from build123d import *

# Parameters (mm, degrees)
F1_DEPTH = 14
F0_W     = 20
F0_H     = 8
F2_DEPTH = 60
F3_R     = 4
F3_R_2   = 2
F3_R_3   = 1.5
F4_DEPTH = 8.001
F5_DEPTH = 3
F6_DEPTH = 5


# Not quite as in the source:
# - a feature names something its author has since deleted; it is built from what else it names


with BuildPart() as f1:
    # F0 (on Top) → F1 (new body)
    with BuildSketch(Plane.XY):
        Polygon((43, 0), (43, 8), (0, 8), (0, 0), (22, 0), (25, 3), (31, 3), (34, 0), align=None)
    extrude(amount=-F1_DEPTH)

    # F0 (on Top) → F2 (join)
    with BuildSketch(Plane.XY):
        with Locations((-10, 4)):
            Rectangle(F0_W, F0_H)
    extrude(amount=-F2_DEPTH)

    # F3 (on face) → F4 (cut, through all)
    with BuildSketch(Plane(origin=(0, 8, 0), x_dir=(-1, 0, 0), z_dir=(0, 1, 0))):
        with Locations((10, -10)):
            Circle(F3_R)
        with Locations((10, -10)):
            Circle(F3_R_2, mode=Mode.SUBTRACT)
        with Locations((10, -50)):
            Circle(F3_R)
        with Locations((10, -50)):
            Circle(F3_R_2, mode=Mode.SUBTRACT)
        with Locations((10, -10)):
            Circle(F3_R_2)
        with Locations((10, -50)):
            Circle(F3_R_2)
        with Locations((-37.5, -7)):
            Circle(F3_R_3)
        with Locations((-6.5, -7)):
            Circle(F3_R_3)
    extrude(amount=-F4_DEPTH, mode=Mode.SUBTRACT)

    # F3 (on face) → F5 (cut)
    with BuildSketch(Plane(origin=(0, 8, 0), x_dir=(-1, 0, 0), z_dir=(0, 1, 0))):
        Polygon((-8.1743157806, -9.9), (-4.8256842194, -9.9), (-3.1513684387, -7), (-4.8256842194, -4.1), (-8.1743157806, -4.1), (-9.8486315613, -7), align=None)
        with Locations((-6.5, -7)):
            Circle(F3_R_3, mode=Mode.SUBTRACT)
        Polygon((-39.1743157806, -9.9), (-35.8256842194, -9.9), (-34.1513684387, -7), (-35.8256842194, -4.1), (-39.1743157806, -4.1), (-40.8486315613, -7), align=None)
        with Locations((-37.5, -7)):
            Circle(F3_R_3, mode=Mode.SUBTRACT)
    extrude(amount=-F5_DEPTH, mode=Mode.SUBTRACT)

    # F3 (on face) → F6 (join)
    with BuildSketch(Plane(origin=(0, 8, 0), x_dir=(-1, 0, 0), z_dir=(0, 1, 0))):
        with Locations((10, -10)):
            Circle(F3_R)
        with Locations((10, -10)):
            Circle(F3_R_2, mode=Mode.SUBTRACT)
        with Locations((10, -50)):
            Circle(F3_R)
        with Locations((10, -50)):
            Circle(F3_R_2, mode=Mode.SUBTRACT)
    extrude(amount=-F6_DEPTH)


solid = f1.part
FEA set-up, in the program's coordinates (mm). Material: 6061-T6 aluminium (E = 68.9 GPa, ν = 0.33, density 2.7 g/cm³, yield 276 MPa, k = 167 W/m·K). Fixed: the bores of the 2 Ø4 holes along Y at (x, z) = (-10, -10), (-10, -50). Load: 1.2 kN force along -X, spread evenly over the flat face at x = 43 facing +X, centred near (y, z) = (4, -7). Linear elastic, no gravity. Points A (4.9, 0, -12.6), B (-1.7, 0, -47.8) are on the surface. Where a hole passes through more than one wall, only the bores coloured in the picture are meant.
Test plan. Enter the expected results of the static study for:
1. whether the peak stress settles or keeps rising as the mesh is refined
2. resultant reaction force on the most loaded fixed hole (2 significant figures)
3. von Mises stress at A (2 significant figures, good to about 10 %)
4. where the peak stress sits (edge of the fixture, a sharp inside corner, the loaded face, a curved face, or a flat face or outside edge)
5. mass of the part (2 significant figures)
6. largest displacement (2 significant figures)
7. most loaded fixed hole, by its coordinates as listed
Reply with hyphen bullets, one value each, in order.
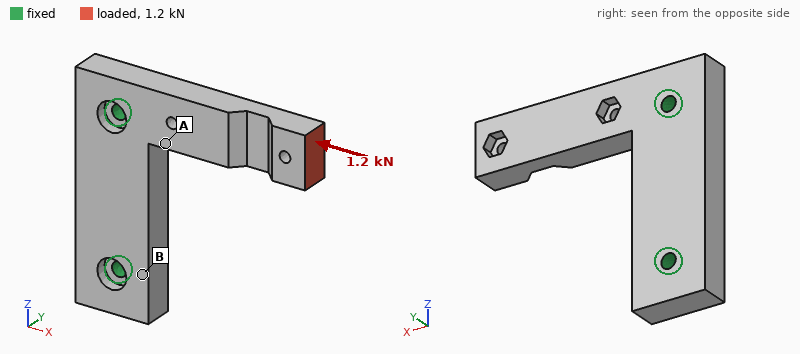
- keeps rising
- 1.3 kN
- 9.7 MPa
- edge of the fixture
- 36 g
- 47 µm
- (-10, -10)
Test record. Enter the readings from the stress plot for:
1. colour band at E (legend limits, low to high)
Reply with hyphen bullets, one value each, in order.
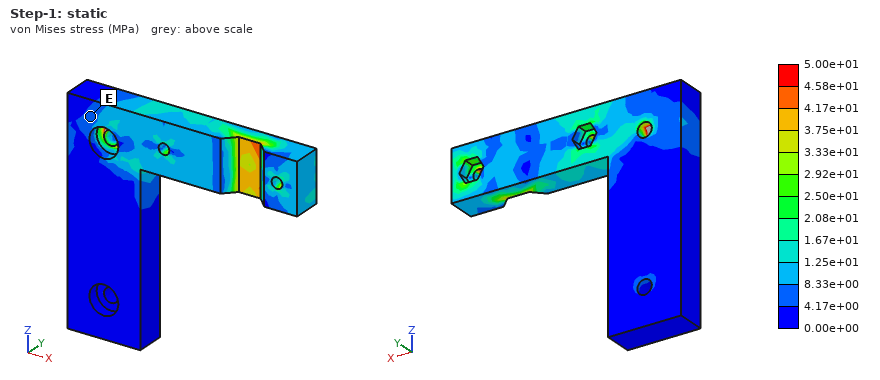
- 4.17e+00 to 8.33e+00 MPa
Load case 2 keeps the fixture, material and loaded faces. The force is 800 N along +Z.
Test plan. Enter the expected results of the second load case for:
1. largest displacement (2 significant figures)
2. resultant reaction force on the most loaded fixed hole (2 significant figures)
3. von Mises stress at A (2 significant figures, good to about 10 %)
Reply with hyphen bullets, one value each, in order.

- 0.37 mm
- 1.0 kN
- 99 MPa
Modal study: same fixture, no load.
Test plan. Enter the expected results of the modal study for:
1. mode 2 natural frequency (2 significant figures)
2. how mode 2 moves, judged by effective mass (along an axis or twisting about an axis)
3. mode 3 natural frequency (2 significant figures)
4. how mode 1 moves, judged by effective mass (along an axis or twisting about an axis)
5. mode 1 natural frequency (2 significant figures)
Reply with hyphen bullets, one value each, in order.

- 4100 Hz
- along Z
- 9900 Hz
- along Y
- 2100 Hz
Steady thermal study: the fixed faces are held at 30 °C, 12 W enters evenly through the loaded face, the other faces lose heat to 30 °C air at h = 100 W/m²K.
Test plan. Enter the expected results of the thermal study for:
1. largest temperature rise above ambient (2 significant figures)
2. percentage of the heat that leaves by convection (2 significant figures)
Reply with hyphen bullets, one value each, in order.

- 33 K
- 32 %
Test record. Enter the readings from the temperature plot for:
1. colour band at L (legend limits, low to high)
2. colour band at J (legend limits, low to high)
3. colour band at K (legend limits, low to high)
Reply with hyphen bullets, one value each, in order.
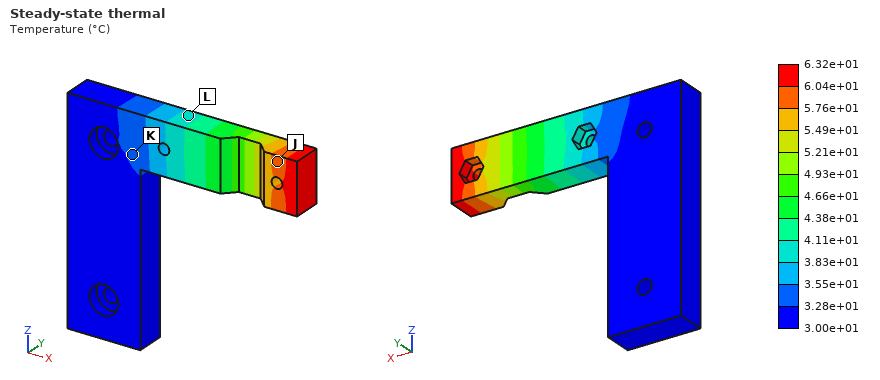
- 3.83e+01 to 4.11e+01 °C
- 5.76e+01 to 6.04e+01 °C
- 3.28e+01 to 3.55e+01 °C
